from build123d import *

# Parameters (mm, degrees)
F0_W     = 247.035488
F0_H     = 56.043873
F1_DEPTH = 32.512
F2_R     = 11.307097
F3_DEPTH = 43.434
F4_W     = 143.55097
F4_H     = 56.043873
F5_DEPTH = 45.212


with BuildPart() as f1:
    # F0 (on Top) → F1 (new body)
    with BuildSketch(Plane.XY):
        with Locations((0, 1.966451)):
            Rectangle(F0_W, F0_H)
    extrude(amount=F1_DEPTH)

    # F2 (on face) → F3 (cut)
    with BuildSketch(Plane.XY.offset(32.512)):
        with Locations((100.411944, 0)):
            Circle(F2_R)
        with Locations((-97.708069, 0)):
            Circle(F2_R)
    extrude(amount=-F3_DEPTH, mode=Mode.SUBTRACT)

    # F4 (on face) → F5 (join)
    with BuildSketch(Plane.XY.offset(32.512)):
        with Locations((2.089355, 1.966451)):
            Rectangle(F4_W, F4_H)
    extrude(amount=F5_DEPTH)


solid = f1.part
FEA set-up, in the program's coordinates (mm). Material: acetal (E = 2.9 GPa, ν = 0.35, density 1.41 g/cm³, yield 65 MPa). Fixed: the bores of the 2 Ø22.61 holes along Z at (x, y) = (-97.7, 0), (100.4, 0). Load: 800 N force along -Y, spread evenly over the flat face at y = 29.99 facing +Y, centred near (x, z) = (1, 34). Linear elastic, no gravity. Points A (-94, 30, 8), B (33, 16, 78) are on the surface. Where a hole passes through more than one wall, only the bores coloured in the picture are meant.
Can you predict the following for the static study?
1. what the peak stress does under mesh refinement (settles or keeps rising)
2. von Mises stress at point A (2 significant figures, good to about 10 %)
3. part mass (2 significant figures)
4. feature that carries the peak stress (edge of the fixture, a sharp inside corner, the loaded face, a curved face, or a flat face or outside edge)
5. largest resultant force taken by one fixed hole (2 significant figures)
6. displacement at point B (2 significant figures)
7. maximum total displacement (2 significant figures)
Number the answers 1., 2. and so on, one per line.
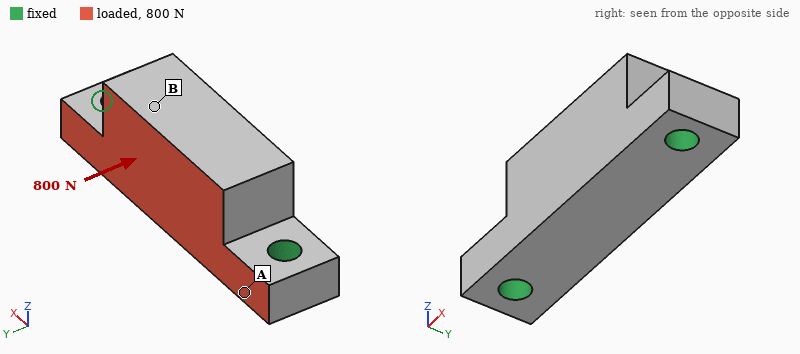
1. keeps rising
2. 0.39 MPa
3. 1.1 kg
4. edge of the fixture
5. 400 N
6. 46 µm
7. 50 µm
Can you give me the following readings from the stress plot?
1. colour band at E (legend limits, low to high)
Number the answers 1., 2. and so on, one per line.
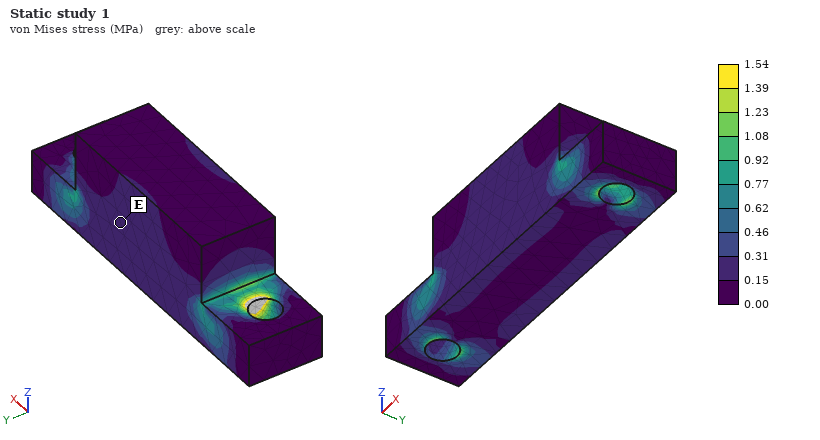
1. 0.15 to 0.31 MPa
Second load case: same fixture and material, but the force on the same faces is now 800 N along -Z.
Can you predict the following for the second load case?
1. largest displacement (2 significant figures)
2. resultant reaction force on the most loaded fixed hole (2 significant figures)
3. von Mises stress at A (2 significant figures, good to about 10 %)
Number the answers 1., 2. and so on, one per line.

1. 55 µm
2. 430 N
3. 0.40 MPa
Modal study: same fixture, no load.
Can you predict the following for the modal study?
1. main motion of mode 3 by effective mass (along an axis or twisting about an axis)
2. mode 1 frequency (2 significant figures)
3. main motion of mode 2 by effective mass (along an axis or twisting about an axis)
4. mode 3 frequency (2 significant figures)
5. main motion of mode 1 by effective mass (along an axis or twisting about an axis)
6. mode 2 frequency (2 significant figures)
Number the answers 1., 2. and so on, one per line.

1. along Y
2. 710 Hz
3. along Z
4. 1500 Hz
5. along Y
6. 1200 Hz
